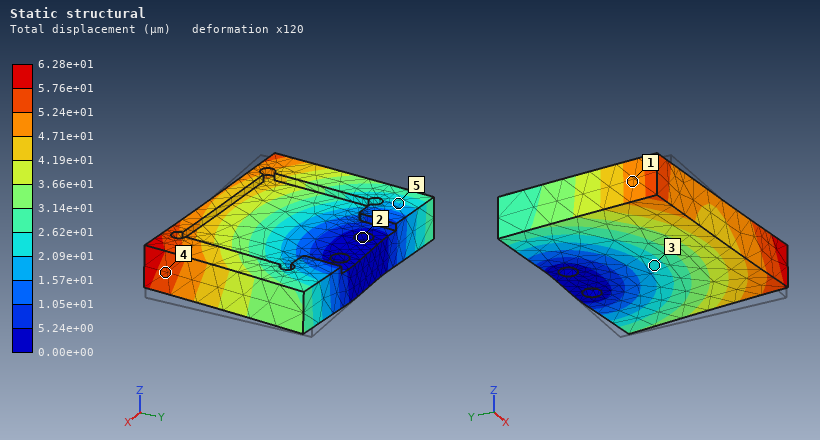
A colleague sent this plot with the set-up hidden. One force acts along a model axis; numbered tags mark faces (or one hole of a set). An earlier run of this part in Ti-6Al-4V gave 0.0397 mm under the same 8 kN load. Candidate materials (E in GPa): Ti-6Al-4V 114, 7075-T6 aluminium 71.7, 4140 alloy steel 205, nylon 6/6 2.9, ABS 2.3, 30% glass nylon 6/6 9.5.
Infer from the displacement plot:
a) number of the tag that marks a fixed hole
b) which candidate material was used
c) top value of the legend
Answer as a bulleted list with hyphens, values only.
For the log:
- 2
- 7075-T6 aluminium
- 6.28e+01 µm
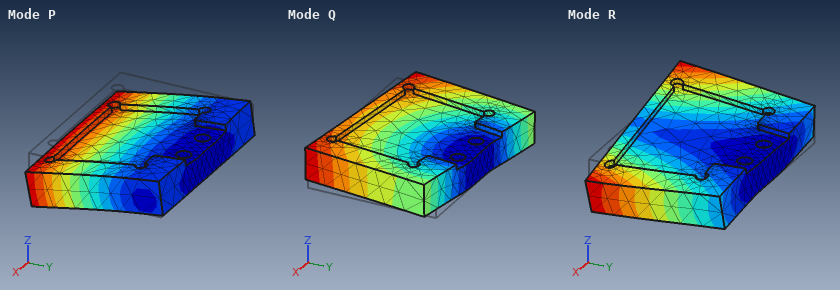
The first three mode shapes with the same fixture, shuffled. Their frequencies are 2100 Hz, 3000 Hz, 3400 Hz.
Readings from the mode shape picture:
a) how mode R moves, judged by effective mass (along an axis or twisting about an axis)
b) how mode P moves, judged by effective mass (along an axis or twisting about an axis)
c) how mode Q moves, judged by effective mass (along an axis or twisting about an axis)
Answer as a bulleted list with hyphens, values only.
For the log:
- twisting about Y
- along Z
- along X
